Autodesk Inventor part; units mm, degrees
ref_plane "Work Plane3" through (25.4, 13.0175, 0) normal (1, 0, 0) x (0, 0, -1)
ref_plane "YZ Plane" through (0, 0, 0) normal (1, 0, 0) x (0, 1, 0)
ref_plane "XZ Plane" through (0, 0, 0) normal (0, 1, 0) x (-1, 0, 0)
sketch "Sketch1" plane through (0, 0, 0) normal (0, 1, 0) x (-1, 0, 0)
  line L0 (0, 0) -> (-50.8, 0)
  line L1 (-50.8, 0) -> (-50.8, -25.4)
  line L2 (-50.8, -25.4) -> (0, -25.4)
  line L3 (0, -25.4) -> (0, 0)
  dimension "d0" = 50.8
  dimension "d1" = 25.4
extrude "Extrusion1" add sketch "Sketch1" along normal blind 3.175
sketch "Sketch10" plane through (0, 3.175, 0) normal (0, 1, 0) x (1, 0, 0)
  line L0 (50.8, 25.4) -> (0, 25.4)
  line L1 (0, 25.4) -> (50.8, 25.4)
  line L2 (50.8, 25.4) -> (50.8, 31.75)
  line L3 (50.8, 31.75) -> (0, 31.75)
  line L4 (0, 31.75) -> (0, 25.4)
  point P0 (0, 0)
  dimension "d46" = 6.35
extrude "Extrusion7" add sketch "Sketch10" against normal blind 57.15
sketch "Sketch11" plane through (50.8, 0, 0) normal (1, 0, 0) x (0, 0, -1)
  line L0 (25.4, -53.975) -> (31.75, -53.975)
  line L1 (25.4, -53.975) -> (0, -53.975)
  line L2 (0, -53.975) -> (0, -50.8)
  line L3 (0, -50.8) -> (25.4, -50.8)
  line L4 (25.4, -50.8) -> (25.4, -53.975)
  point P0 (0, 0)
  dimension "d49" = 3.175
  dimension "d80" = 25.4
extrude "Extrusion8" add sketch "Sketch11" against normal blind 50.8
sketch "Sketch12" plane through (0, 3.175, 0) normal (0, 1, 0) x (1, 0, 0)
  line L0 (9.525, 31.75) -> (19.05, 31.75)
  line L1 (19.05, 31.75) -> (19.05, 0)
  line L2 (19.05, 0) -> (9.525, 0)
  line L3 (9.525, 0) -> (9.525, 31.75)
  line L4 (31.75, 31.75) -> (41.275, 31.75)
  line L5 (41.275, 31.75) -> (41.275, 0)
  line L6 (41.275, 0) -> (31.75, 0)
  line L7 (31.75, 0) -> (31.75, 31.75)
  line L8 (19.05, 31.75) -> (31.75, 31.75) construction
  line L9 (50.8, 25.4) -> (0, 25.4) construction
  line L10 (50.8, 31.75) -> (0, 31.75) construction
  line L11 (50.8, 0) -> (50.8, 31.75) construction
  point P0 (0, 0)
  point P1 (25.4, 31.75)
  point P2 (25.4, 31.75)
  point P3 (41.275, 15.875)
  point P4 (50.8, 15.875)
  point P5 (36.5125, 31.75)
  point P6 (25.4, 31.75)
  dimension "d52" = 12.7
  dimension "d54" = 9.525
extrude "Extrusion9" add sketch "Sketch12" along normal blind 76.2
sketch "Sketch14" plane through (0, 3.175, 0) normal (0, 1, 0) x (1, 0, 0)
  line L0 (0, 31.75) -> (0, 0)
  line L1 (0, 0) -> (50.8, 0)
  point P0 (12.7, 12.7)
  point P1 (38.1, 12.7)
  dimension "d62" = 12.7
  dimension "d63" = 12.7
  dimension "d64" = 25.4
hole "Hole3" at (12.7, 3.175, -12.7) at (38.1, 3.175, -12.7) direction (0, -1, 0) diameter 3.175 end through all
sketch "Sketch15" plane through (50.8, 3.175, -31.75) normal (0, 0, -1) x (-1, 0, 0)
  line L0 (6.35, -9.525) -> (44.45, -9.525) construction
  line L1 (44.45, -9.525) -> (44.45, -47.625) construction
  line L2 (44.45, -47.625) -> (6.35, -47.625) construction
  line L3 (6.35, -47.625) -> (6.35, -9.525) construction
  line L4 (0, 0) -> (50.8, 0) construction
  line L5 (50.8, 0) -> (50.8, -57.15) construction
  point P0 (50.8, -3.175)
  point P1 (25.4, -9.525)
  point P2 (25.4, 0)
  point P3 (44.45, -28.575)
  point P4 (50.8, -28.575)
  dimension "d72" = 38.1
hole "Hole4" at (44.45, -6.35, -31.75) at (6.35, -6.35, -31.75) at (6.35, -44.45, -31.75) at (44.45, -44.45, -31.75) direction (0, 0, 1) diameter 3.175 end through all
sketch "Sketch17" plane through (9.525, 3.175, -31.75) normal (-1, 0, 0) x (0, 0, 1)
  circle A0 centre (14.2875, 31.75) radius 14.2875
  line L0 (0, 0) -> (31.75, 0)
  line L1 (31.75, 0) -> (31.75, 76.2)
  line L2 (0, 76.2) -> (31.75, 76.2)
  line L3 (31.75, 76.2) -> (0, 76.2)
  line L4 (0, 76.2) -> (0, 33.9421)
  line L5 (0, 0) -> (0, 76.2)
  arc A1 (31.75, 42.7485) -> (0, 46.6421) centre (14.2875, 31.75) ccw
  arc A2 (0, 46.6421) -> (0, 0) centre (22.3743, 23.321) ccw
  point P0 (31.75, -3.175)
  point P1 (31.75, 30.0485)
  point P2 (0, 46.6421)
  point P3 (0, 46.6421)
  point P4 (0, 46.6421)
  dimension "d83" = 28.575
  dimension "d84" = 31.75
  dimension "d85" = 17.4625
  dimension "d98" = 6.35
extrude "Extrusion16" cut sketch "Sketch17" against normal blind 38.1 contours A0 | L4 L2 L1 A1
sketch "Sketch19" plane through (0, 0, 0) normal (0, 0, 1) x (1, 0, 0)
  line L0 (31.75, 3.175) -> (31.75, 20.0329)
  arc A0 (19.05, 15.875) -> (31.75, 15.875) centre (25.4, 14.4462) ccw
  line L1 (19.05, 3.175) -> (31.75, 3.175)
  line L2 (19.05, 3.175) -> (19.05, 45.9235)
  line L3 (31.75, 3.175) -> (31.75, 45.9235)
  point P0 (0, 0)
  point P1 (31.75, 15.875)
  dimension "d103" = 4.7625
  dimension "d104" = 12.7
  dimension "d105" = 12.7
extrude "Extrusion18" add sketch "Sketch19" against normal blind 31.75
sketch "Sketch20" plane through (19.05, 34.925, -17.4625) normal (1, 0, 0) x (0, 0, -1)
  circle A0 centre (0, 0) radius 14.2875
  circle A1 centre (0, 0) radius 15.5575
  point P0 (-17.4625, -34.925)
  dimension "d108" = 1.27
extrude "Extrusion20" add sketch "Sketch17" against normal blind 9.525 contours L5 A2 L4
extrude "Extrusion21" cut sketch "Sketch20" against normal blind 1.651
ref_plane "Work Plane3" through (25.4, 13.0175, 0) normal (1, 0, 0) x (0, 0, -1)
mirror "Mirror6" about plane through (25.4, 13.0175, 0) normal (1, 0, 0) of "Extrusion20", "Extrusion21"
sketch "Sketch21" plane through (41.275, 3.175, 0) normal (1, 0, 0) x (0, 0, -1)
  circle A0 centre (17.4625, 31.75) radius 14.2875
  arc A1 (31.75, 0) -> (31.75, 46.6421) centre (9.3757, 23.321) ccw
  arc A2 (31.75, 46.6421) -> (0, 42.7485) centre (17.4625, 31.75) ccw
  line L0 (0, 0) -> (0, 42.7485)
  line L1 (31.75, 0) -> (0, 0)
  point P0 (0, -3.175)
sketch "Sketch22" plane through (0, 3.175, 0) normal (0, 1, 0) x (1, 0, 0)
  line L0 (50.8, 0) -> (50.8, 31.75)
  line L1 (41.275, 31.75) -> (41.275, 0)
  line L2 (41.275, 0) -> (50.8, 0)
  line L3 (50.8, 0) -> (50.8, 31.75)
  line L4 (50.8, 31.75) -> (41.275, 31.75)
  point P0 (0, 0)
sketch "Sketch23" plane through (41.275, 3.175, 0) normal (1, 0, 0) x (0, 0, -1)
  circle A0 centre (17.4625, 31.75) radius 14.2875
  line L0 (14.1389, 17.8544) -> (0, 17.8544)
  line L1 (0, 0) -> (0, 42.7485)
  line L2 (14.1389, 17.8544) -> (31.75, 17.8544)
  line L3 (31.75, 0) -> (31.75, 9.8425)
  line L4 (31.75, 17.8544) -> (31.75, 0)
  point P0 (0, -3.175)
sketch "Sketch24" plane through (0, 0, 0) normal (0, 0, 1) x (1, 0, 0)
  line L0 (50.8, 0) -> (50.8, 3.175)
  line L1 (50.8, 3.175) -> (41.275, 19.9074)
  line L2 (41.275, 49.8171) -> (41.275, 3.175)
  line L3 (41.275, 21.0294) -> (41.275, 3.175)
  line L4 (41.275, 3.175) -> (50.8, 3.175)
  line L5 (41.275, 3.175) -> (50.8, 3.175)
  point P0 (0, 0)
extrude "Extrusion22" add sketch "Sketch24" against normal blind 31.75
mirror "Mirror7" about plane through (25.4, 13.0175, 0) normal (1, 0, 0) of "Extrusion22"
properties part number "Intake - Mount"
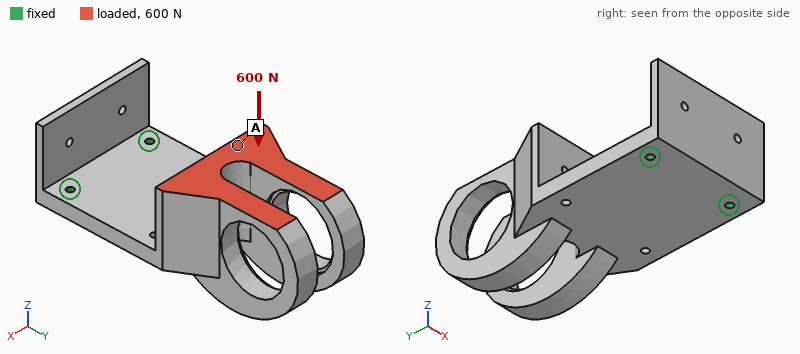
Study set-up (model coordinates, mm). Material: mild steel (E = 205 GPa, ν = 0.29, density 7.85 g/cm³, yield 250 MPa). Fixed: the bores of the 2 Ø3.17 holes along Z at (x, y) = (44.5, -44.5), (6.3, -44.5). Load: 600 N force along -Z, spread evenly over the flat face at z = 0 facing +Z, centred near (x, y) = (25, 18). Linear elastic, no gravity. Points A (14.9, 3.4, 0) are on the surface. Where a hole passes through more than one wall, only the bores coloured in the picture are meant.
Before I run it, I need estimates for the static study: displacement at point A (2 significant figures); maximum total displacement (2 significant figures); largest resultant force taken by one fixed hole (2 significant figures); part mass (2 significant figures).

0.24 mm
0.47 mm
310 N
450 g
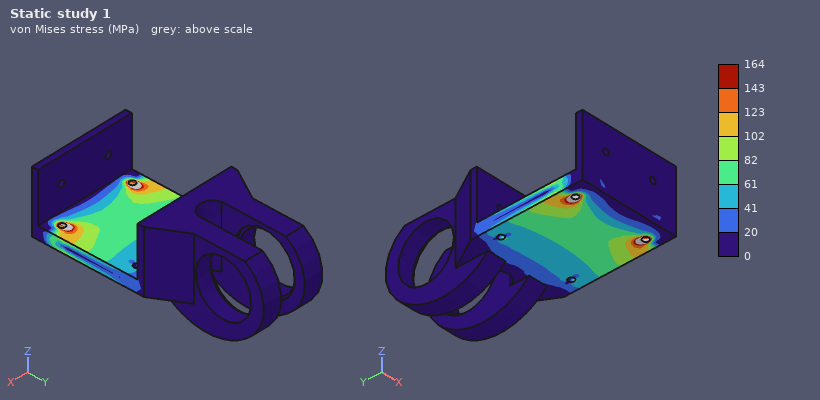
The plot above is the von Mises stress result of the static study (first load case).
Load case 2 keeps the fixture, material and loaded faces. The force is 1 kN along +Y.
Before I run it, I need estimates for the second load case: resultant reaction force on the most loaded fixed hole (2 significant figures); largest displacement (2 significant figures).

520 N
0.52 mm
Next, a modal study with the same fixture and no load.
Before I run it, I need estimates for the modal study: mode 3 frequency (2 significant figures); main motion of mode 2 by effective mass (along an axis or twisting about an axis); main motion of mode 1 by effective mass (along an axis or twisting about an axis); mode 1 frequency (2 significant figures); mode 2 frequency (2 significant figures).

2500 Hz
along X
along Z
410 Hz
1500 Hz
